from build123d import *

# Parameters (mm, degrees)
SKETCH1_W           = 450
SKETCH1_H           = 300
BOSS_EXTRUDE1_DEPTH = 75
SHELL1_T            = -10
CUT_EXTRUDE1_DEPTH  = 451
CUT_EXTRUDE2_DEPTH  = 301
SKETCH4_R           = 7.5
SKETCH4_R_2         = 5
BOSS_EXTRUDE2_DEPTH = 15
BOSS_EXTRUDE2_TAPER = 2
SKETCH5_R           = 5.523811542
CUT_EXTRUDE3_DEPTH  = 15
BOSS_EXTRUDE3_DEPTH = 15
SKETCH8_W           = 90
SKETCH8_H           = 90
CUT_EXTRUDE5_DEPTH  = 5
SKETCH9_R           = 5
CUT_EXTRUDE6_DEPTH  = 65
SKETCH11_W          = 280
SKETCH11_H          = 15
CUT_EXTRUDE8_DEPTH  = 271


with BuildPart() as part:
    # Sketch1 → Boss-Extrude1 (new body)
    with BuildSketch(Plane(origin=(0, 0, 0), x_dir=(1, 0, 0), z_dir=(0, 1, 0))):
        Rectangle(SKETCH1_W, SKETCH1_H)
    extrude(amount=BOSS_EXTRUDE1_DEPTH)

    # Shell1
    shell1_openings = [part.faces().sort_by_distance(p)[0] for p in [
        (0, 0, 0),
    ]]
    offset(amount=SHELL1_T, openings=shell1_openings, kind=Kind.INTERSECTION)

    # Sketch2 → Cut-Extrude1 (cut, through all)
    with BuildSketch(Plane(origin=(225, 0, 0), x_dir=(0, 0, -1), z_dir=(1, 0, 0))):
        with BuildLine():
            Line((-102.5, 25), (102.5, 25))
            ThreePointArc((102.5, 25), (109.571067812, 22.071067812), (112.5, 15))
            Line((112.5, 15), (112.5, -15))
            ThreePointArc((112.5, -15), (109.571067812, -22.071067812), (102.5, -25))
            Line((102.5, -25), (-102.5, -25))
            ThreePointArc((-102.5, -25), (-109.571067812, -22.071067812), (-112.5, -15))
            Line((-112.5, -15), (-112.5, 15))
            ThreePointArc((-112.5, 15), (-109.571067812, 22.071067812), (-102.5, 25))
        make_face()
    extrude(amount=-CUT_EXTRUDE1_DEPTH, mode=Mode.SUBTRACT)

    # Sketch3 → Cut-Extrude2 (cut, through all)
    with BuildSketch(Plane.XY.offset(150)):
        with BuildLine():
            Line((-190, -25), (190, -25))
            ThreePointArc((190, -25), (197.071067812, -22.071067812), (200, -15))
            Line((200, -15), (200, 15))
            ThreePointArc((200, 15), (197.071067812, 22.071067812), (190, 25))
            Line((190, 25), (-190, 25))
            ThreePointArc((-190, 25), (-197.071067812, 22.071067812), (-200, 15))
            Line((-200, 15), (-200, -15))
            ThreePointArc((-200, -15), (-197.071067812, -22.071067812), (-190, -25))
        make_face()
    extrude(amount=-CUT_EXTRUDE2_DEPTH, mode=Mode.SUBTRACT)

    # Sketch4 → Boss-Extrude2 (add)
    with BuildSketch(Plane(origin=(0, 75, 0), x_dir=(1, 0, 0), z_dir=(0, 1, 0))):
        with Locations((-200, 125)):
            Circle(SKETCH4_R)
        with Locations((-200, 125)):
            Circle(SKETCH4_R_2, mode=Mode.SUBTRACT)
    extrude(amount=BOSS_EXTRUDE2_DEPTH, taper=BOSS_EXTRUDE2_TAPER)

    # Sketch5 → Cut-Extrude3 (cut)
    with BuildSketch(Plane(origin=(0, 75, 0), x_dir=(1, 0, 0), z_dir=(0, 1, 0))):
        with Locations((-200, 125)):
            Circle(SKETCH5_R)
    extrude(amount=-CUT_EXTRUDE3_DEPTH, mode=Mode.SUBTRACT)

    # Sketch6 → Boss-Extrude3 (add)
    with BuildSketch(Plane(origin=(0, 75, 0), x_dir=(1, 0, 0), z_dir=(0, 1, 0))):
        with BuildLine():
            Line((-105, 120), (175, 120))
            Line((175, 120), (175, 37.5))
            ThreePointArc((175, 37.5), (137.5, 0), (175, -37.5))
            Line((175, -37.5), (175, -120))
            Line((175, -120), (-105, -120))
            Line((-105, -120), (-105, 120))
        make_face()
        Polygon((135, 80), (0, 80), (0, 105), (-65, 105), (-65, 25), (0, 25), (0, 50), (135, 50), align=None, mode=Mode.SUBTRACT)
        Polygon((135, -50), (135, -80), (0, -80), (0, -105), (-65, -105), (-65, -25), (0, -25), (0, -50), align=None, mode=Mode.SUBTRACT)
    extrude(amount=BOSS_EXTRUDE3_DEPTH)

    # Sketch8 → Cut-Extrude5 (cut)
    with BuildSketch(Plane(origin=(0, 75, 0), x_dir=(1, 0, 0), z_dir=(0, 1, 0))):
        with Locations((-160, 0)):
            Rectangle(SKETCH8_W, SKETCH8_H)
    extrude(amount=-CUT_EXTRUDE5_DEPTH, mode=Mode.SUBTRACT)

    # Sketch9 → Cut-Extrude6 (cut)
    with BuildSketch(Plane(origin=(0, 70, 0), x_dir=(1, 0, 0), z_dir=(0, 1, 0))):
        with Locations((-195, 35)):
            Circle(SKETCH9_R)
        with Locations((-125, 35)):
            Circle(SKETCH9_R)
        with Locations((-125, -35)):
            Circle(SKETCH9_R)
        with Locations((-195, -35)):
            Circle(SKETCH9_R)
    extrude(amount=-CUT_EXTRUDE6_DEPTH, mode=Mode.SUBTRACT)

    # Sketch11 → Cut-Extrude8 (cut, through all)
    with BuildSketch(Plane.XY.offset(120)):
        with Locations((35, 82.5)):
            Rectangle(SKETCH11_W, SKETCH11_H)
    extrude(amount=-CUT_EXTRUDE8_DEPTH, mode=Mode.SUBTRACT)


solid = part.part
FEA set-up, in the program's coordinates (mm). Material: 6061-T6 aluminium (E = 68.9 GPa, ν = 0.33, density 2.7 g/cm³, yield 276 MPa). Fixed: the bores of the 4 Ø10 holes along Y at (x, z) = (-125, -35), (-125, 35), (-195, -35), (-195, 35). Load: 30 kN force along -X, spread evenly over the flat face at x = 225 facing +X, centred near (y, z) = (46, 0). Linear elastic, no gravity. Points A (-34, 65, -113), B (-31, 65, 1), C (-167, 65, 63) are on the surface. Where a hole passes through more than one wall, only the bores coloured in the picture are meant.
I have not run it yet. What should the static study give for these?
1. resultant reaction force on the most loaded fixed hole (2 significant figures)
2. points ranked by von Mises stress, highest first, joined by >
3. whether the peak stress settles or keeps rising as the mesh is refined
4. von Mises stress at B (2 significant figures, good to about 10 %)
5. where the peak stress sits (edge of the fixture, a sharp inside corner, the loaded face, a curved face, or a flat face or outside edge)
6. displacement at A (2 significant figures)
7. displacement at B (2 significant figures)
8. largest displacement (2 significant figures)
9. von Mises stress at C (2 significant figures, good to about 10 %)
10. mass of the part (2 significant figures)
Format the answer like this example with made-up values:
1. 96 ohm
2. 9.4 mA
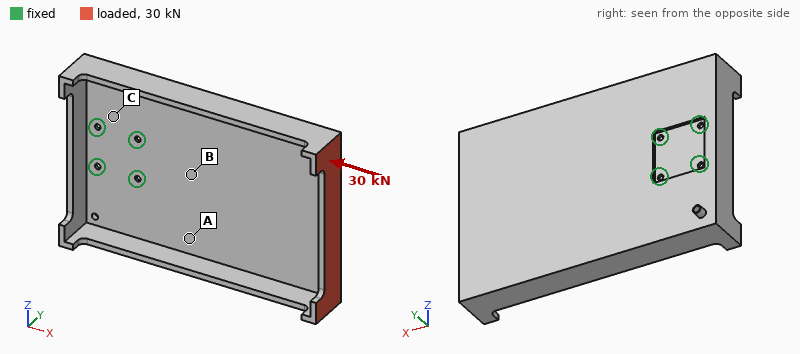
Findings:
1. 12 kN
2. C > B > A
3. keeps rising
4. 30 MPa
5. edge of the fixture
6. 1.3 mm
7. 0.94 mm
8. 5.4 mm
9. 53 MPa
10. 5.3 kg
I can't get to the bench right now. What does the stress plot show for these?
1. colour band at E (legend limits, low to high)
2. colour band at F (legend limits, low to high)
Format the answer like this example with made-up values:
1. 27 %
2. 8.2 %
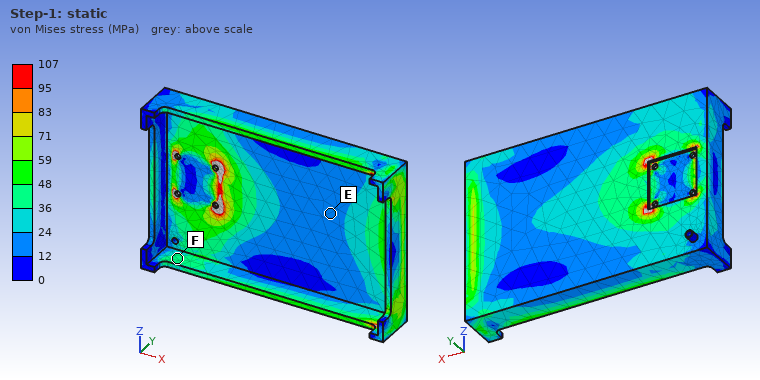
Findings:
1. 12 to 24 MPa
2. 36 to 48 MPa
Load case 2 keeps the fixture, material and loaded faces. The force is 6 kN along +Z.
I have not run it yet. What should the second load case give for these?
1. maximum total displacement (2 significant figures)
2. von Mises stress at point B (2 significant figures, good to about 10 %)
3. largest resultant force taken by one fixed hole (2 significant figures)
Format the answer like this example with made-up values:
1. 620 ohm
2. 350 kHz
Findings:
1. 2.1 mm
2. 23 MPa
3. 13 kN
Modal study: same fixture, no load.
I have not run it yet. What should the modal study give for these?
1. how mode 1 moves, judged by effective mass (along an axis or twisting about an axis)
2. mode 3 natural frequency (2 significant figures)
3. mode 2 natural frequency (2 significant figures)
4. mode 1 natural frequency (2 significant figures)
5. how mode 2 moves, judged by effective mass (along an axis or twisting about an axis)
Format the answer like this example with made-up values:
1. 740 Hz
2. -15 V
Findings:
1. along Y
2. 470 Hz
3. 130 Hz
4. 75 Hz
5. twisting about X
